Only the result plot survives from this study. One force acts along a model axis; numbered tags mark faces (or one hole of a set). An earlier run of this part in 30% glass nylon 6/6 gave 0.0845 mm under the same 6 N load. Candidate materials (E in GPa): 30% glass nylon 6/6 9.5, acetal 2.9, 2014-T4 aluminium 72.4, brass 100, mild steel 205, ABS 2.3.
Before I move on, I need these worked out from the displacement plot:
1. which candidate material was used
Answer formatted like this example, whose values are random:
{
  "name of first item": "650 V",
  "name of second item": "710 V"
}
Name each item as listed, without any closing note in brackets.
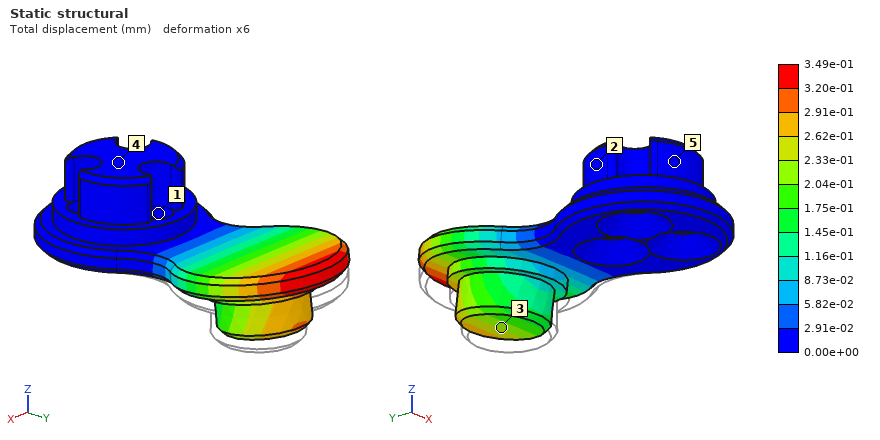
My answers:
{
  "which candidate material was used": "ABS"
}
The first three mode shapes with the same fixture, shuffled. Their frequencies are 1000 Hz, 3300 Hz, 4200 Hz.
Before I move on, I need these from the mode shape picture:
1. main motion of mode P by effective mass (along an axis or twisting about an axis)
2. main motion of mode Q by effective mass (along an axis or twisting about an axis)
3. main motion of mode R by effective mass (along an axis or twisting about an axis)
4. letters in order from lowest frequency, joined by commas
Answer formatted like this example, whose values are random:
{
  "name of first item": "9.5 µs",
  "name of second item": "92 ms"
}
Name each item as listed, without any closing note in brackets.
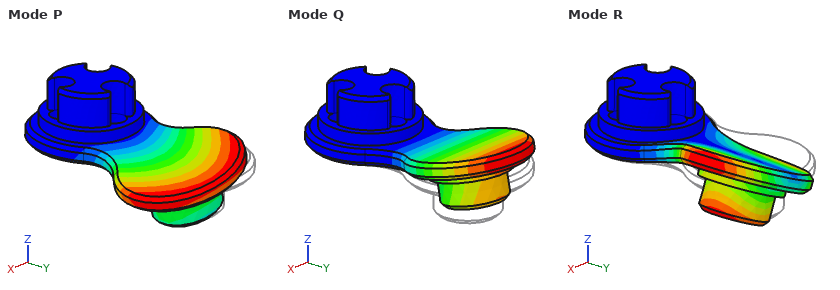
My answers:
{
  "main motion of mode P by effective mass": "along X",
  "main motion of mode Q by effective mass": "along Z",
  "main motion of mode R by effective mass": "along X",
  "letters in order from lowest frequency, joined by commas": "Q, R, P"
}
